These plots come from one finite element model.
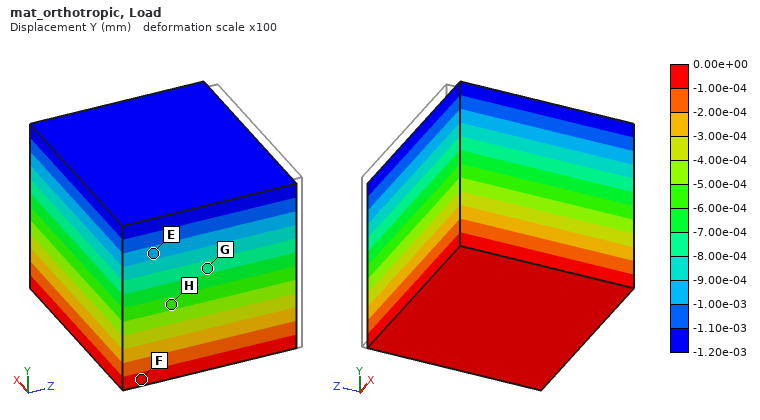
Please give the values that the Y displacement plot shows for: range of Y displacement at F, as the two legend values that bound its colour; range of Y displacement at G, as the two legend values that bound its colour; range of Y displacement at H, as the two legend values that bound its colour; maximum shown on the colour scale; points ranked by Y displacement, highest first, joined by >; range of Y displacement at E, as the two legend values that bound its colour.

-1.00e-04 to 0.00e+00 mm
-8.00e-04 to -7.00e-04 mm
-6.00e-04 to -5.00e-04 mm
0.00e+00 mm
F > H > G > E
-1.00e-03 to -9.00e-04 mm
